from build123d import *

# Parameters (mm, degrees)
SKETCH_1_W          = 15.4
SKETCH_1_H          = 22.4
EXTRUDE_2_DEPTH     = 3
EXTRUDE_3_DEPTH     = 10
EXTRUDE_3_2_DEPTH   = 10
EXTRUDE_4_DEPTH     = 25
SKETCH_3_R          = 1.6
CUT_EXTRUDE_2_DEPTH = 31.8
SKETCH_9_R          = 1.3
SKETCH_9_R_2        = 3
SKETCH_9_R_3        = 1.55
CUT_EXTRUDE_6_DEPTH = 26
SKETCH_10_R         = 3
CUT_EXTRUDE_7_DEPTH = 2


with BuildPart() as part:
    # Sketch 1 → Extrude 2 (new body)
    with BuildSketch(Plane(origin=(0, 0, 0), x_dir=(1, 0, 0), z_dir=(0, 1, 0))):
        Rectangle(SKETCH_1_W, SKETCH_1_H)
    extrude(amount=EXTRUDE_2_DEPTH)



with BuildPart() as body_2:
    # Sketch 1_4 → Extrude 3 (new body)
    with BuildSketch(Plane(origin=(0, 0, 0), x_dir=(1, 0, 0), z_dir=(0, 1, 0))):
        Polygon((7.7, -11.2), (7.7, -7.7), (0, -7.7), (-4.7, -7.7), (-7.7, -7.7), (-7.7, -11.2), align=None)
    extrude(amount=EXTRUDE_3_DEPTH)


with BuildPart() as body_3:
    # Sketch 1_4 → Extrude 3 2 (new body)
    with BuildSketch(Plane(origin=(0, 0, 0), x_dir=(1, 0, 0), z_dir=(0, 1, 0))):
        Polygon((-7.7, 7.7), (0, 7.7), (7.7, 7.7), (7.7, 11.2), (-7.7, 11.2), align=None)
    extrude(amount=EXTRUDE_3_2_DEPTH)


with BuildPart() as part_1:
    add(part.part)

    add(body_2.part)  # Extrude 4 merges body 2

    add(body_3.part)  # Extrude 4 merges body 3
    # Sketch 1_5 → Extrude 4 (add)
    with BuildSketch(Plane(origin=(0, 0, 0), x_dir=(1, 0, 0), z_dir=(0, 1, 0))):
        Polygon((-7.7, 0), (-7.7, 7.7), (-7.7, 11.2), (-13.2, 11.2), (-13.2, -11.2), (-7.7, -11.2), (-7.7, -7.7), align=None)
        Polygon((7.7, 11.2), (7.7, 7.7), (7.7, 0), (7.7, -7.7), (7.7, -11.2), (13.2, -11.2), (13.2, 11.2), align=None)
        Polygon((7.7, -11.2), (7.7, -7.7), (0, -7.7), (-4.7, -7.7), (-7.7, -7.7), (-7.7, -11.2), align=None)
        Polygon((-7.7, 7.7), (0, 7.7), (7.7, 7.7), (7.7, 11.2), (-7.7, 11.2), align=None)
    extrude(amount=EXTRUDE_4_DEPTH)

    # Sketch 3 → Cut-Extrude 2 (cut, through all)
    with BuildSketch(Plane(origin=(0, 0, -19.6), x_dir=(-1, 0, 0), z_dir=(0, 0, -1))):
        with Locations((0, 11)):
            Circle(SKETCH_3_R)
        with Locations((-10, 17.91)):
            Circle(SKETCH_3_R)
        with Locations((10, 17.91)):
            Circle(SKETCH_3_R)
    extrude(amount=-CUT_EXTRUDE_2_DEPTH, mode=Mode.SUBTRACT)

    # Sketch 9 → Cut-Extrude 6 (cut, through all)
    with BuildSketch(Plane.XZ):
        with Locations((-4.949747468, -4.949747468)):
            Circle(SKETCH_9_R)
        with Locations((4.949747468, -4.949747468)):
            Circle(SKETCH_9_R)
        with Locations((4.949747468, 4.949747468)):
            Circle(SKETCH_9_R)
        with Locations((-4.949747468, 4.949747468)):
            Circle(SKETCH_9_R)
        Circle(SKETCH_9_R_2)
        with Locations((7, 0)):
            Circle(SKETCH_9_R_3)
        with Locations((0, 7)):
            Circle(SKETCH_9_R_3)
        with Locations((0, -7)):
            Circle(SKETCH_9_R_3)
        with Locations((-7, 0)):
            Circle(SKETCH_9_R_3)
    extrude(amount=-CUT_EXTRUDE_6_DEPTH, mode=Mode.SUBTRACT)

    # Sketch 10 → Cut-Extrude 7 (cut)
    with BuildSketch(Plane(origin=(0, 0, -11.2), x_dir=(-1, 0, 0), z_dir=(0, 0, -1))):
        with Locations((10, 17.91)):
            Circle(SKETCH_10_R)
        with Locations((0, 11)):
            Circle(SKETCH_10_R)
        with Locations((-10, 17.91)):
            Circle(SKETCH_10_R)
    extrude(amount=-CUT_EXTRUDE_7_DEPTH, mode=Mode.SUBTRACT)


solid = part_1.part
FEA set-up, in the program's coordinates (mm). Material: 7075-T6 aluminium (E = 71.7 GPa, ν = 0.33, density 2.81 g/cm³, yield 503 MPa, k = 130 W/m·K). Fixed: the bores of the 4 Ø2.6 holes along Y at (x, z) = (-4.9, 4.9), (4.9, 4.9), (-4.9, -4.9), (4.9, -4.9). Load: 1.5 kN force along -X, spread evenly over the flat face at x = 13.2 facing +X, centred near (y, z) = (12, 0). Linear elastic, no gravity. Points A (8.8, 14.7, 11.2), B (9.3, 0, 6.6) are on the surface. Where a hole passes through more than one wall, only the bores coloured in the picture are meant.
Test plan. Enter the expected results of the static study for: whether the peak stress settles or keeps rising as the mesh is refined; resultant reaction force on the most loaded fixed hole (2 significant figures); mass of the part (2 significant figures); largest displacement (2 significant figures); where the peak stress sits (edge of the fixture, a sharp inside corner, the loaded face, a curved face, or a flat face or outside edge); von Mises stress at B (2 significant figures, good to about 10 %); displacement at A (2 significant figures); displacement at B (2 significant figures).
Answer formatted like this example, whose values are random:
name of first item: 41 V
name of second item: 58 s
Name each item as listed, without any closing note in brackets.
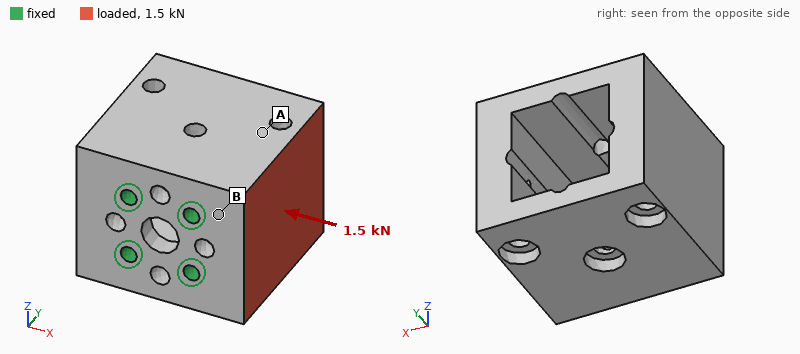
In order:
whether the peak stress settles or keeps rising as the mesh is refined: keeps rising
resultant reaction force on the most loaded fixed hole: 760 N
mass of the part: 24 g
largest displacement: 36 µm
where the peak stress sits: edge of the fixture
von Mises stress at B: 22 MPa
displacement at A: 19 µm
displacement at B: 7.1 µm
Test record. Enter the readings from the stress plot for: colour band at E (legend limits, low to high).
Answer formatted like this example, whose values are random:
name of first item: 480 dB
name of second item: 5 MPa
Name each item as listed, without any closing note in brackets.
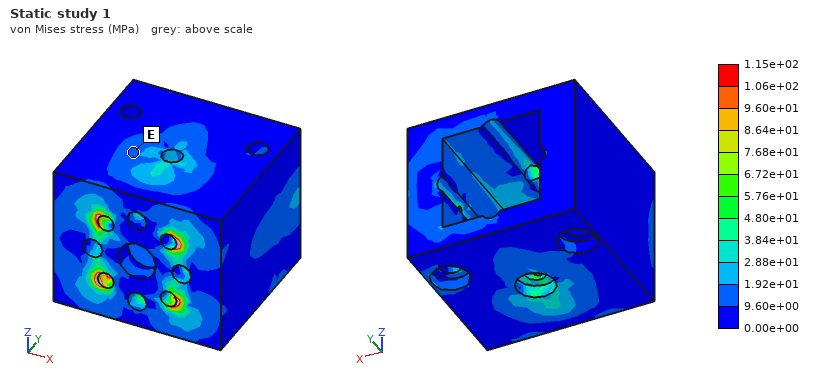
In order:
colour band at E: 9.60e+00 to 1.92e+01 MPa
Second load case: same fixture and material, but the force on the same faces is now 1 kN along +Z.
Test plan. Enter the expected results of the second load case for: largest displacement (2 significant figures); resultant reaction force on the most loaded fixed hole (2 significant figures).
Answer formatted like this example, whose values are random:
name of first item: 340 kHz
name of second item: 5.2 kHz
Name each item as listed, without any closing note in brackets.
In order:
largest displacement: 26 µm
resultant reaction force on the most loaded fixed hole: 830 N
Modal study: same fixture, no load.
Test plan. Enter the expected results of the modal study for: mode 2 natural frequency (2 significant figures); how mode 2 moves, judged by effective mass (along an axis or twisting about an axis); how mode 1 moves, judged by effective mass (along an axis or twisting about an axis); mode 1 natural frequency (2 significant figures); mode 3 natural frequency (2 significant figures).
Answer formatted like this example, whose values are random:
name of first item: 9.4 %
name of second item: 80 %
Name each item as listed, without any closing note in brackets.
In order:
mode 2 natural frequency: 9000 Hz
how mode 2 moves, judged by effective mass: along Z
how mode 1 moves, judged by effective mass: along X
mode 1 natural frequency: 8300 Hz
mode 3 natural frequency: 16 kHz
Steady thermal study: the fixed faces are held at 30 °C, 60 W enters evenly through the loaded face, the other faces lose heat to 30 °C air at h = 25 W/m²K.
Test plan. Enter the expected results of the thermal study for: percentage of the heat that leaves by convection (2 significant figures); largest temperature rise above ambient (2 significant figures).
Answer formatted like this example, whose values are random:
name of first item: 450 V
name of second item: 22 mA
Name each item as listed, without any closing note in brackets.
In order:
percentage of the heat that leaves by convection: 3.7 %
largest temperature rise above ambient: 43 K
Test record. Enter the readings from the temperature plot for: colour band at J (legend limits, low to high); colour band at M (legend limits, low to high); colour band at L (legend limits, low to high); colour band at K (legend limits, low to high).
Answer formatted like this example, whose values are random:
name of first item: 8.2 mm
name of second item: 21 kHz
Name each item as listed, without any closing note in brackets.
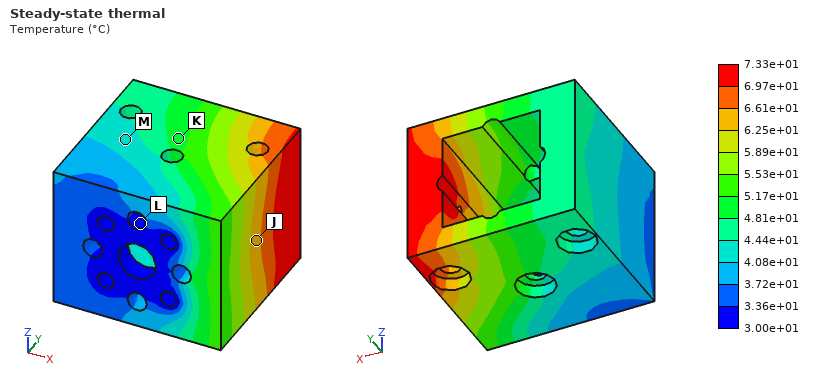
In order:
colour band at J: 6.25e+01 to 6.61e+01 °C
colour band at M: 4.08e+01 to 4.44e+01 °C
colour band at L: 3.00e+01 to 3.36e+01 °C
colour band at K: 4.81e+01 to 5.17e+01 °C
